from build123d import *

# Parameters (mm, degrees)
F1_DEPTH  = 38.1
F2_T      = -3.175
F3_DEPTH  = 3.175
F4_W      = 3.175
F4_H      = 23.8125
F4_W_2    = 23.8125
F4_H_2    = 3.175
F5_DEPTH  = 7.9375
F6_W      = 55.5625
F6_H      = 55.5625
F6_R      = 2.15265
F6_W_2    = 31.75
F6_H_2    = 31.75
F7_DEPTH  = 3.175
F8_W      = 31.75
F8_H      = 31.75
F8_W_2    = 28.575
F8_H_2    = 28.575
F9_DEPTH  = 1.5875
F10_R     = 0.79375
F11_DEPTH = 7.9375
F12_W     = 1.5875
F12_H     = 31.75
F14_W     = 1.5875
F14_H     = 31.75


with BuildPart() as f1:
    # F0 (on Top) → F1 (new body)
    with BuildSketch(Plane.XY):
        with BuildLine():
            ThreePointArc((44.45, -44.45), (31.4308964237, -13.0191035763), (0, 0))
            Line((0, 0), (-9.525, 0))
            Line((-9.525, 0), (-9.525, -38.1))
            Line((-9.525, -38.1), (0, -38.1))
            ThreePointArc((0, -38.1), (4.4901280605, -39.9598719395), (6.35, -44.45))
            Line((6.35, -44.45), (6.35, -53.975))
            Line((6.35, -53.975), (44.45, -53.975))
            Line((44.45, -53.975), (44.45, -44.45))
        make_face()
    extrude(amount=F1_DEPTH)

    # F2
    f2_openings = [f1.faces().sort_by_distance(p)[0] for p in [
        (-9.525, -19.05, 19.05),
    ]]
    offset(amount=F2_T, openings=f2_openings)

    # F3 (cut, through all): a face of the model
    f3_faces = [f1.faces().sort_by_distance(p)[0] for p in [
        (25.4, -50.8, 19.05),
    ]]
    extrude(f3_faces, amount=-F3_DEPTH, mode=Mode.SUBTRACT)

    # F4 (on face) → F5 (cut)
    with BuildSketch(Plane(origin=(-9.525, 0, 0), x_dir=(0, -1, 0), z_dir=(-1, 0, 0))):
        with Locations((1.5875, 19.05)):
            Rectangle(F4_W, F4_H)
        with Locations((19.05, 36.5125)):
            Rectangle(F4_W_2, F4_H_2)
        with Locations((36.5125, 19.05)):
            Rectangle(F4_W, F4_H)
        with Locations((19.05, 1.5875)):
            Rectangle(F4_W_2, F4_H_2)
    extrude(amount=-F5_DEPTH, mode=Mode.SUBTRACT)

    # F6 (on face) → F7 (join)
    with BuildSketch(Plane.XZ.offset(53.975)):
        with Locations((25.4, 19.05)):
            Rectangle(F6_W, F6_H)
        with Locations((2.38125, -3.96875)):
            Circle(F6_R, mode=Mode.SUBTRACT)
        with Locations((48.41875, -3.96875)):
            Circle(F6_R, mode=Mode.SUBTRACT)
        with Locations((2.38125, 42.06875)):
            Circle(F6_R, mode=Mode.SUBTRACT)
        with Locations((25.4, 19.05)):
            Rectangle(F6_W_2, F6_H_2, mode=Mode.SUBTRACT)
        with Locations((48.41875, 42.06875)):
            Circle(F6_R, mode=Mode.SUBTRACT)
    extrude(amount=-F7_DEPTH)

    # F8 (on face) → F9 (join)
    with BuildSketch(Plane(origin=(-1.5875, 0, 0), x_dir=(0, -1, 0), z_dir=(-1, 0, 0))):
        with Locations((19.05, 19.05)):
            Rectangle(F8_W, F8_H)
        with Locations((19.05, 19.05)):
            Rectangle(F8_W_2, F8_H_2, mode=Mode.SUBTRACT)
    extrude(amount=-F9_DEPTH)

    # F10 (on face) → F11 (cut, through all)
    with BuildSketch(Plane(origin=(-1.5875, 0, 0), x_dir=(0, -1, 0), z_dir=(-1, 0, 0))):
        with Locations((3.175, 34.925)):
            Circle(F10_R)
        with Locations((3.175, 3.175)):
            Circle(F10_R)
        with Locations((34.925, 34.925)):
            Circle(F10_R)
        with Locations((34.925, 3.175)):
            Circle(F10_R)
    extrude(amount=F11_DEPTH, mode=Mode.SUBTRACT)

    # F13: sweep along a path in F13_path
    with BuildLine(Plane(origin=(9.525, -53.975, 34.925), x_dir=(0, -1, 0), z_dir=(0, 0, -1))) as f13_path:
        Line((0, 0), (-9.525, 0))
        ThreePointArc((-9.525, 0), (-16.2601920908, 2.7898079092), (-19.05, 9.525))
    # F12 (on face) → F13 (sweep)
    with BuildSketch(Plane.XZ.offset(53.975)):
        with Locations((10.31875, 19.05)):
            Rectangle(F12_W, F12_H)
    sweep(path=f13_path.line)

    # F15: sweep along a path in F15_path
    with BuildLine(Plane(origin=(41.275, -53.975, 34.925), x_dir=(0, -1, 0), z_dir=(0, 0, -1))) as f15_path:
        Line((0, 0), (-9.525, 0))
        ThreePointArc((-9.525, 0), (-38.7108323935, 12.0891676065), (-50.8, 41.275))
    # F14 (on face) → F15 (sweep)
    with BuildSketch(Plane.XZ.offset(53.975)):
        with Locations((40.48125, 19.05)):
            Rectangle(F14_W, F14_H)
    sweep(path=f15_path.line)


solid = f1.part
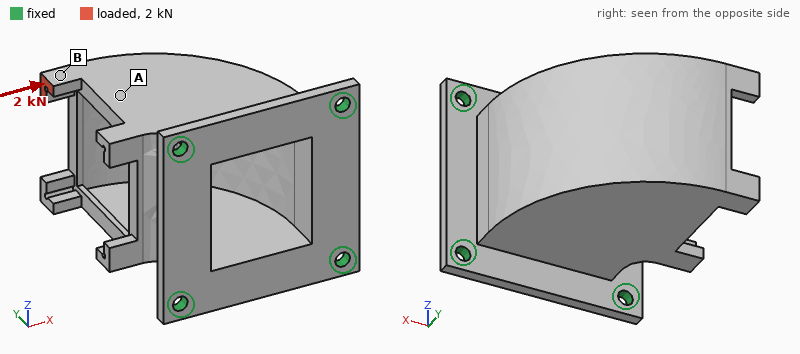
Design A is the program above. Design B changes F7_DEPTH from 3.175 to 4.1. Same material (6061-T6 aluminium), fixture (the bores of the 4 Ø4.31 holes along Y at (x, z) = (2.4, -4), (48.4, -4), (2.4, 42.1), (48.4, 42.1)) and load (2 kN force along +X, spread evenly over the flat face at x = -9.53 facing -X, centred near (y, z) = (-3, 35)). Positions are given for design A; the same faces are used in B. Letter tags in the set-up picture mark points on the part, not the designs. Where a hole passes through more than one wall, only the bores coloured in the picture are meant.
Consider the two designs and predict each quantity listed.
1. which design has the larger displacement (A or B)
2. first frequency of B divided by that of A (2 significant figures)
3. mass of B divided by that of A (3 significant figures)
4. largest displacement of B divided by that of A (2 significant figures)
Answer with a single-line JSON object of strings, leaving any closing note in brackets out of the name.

{"which design has the larger displacement": "A", "first frequency of B divided by that of A": "1.1", "mass of B divided by that of A": "1.04", "largest displacement of B divided by that of A": "0.84"}
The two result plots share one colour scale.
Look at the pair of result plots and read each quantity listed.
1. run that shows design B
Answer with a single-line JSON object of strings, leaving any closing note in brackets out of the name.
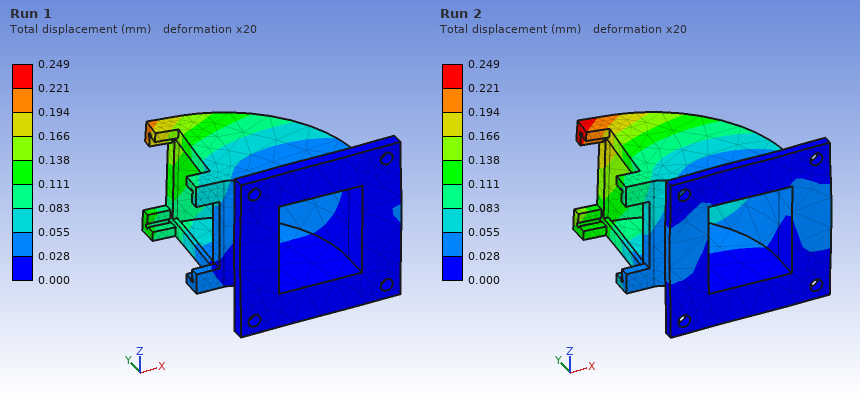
{"run that shows design B": "Run 1"}
